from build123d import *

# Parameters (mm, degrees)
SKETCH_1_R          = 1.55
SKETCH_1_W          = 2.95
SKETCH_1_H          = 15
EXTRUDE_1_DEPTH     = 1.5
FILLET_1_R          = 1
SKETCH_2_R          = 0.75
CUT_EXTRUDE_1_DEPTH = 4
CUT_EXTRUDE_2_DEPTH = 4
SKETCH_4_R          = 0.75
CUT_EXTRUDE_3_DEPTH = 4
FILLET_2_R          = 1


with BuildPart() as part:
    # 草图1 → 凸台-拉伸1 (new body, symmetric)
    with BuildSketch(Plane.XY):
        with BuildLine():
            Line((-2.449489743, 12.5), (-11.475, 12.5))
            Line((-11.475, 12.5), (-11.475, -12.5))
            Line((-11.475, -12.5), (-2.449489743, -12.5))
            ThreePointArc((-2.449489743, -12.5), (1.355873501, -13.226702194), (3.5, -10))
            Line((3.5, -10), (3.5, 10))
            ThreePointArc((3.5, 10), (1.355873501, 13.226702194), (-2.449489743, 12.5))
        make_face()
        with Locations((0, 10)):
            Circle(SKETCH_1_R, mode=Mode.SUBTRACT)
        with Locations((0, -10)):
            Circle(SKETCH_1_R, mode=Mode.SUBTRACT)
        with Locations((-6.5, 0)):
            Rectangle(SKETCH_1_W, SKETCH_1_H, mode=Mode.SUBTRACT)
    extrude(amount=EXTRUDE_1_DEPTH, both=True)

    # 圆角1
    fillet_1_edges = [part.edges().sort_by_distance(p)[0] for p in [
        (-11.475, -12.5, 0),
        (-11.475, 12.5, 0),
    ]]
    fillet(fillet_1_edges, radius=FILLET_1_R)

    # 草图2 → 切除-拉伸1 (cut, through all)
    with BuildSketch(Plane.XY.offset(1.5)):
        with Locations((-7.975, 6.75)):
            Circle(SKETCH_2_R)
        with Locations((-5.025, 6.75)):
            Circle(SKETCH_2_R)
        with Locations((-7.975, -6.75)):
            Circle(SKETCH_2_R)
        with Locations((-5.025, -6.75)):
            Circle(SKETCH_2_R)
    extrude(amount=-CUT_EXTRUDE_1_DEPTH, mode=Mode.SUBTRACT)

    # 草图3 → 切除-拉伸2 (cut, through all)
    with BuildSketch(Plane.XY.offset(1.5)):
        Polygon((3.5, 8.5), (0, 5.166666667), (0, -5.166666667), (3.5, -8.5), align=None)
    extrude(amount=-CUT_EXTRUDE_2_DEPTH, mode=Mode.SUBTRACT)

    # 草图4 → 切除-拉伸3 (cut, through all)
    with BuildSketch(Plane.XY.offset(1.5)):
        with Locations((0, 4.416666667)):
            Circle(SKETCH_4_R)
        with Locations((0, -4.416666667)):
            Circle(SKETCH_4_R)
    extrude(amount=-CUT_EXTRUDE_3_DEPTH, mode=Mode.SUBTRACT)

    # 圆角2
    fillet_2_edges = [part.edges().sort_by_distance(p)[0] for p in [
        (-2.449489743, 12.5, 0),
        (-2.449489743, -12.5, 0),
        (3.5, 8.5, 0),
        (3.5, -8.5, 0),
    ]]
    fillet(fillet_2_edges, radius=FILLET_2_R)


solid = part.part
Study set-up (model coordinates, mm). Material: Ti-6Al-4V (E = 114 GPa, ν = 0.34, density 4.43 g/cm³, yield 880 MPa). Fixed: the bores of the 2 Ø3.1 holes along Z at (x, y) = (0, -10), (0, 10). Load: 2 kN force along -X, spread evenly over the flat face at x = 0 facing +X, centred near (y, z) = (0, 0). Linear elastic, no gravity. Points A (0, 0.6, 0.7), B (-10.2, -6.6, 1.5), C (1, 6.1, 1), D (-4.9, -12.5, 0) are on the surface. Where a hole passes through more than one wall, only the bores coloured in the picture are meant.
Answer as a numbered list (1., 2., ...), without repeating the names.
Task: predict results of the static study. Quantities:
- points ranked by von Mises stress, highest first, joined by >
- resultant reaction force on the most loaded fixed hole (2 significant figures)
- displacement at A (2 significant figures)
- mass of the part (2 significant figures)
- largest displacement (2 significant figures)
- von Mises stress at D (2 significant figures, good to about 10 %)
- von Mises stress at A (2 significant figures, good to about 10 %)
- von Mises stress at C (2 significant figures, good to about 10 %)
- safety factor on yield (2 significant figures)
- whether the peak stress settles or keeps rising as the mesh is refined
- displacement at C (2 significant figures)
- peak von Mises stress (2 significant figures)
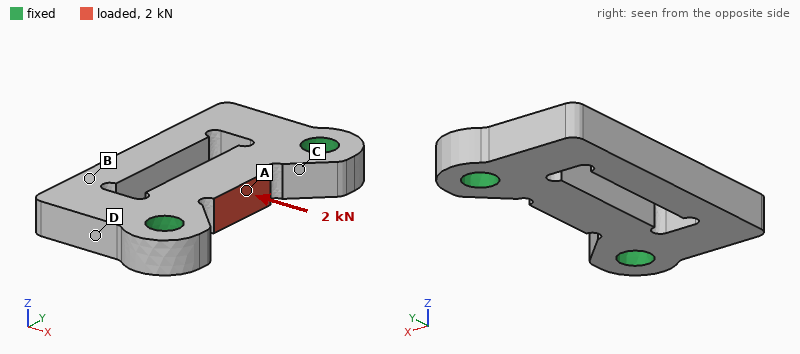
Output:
1. A > C > D > B
2. 1.2 kN
3. 24 µm
4. 3.5 g
5. 24 µm
6. 50 MPa
7. 190 MPa
8. 140 MPa
9. 2.4
10. settles
11. 5.4 µm
12. 370 MPa
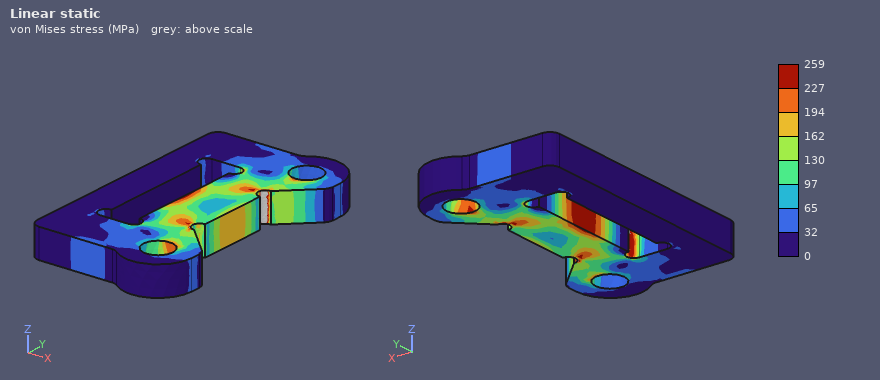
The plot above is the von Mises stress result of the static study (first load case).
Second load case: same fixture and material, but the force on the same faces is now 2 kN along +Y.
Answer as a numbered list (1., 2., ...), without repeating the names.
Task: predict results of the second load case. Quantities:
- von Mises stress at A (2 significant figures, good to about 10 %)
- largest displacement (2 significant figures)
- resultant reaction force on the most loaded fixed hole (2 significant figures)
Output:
1. 160 MPa
2. 14 µm
3. 1.0 kN
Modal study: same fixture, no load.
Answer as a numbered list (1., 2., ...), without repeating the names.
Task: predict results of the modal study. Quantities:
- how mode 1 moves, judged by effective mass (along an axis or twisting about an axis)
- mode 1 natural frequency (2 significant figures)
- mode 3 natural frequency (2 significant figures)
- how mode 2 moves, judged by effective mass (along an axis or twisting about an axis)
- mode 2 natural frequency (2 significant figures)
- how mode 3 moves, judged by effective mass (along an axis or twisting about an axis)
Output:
1. along Z
2. 14 kHz
3. 28 kHz
4. twisting about X
5. 24 kHz
6. along Y
